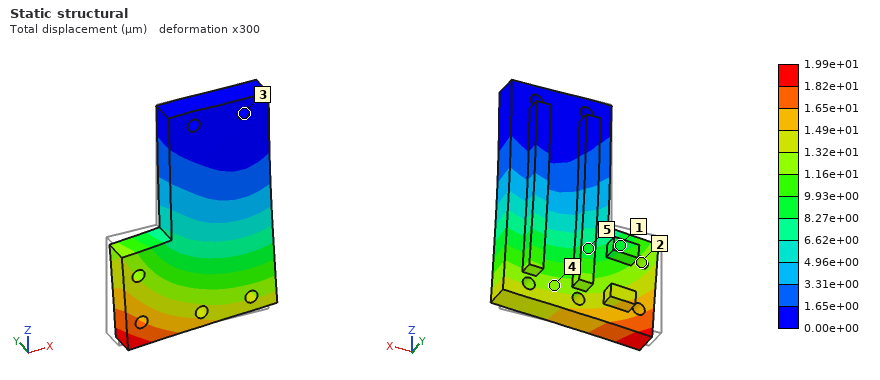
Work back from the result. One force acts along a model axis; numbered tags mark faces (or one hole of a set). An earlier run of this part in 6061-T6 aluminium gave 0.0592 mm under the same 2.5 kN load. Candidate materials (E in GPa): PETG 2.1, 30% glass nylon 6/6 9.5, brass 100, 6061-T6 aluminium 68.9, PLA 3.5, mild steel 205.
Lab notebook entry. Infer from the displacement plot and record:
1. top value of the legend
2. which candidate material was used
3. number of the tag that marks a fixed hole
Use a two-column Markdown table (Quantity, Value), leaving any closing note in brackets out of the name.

| Quantity | Value |
|---|---|
| top value of the legend | 1.99e+01 µm |
| which candidate material was used | mild steel |
| number of the tag that marks a fixed hole | 3 |
